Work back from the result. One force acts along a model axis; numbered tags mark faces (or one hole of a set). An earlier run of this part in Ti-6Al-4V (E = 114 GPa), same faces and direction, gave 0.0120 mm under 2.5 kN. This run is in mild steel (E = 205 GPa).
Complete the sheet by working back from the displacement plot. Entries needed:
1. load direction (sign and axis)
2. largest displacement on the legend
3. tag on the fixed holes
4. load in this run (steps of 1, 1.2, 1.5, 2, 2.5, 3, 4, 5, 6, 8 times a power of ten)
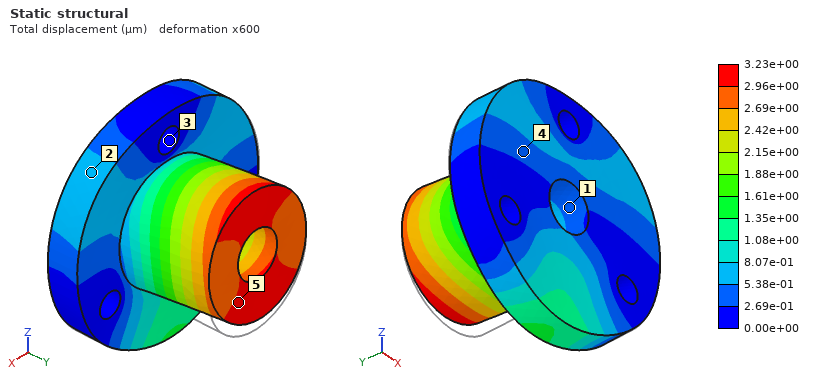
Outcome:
+Z
3.23e+00 µm
3
1.2 kN
